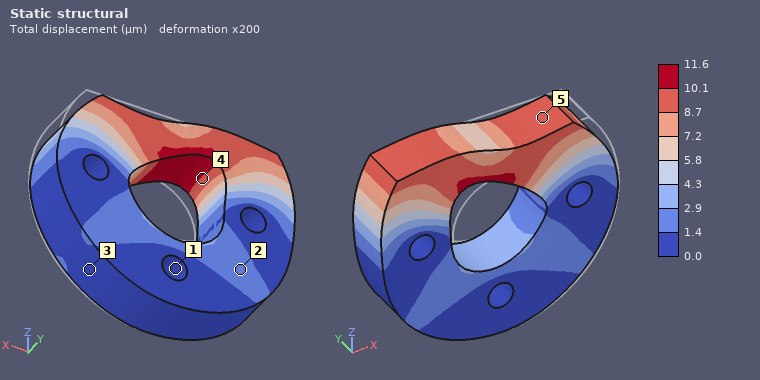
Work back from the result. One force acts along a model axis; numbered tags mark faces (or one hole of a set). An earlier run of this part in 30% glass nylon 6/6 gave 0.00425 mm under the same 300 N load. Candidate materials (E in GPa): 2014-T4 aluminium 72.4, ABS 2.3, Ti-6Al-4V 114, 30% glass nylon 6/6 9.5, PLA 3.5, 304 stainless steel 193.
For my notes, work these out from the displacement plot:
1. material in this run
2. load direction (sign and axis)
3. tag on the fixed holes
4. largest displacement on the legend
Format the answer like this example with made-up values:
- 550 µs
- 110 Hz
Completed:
- PLA
- -X
- 1
- 11.6 µm
